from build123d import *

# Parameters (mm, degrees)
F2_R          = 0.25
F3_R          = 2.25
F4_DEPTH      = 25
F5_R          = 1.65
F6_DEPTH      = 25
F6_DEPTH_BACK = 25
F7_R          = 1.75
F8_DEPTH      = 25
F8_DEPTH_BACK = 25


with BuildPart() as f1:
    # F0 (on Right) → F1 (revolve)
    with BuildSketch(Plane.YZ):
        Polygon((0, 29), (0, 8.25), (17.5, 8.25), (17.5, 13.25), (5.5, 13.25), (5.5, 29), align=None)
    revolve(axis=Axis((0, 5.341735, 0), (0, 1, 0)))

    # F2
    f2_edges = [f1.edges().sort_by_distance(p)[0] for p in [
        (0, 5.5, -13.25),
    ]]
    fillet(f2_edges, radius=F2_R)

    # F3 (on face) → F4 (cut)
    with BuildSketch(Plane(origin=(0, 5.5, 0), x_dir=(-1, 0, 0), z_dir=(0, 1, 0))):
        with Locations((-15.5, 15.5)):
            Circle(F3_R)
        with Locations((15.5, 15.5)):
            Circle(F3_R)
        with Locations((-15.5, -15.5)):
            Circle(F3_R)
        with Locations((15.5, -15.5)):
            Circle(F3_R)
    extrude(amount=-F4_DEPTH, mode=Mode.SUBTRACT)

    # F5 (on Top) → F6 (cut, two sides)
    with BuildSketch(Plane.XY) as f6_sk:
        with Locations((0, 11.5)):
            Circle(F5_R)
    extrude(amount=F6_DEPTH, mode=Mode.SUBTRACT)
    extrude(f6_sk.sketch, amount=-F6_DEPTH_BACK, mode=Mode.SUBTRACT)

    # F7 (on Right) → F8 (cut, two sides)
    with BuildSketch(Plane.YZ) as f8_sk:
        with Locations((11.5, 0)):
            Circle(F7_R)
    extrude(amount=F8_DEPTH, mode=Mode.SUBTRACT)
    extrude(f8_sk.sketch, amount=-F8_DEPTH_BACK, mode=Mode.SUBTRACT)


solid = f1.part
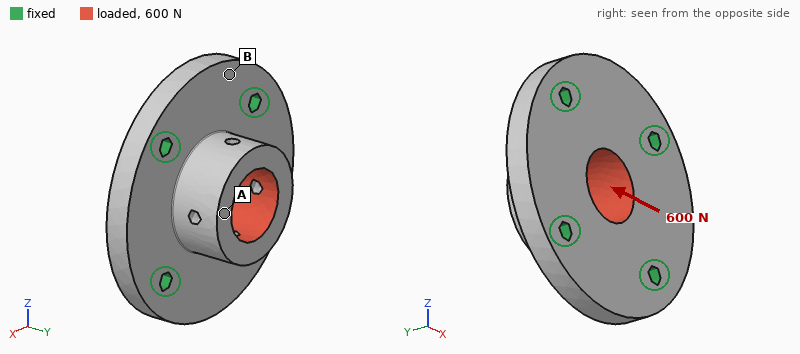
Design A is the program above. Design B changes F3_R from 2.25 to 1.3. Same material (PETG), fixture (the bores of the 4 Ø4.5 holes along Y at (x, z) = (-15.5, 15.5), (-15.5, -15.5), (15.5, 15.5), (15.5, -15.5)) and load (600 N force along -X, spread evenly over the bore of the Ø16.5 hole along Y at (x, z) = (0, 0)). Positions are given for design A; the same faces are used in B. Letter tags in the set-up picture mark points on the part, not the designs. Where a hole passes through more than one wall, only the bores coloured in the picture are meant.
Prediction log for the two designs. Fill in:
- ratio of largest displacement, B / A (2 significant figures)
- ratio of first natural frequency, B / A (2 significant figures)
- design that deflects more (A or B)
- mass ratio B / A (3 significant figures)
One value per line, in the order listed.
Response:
1.1
0.86
B
1.01
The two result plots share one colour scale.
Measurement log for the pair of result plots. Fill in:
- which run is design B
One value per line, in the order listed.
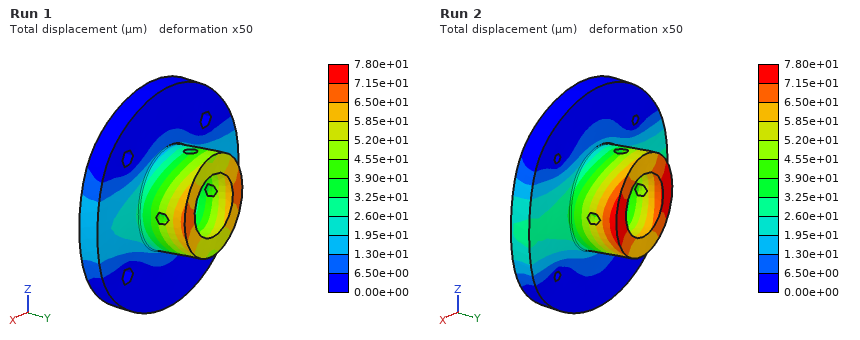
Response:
Run 2
